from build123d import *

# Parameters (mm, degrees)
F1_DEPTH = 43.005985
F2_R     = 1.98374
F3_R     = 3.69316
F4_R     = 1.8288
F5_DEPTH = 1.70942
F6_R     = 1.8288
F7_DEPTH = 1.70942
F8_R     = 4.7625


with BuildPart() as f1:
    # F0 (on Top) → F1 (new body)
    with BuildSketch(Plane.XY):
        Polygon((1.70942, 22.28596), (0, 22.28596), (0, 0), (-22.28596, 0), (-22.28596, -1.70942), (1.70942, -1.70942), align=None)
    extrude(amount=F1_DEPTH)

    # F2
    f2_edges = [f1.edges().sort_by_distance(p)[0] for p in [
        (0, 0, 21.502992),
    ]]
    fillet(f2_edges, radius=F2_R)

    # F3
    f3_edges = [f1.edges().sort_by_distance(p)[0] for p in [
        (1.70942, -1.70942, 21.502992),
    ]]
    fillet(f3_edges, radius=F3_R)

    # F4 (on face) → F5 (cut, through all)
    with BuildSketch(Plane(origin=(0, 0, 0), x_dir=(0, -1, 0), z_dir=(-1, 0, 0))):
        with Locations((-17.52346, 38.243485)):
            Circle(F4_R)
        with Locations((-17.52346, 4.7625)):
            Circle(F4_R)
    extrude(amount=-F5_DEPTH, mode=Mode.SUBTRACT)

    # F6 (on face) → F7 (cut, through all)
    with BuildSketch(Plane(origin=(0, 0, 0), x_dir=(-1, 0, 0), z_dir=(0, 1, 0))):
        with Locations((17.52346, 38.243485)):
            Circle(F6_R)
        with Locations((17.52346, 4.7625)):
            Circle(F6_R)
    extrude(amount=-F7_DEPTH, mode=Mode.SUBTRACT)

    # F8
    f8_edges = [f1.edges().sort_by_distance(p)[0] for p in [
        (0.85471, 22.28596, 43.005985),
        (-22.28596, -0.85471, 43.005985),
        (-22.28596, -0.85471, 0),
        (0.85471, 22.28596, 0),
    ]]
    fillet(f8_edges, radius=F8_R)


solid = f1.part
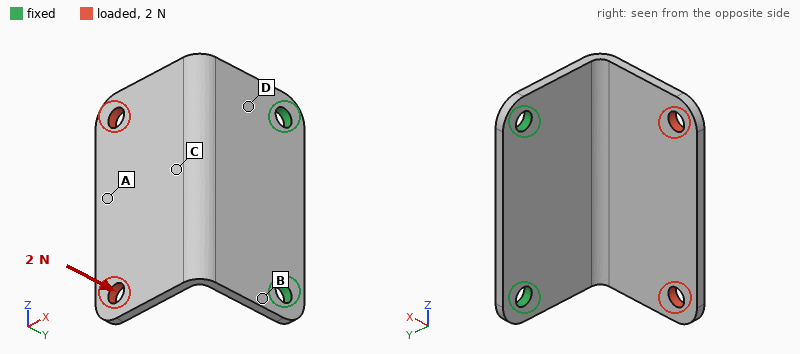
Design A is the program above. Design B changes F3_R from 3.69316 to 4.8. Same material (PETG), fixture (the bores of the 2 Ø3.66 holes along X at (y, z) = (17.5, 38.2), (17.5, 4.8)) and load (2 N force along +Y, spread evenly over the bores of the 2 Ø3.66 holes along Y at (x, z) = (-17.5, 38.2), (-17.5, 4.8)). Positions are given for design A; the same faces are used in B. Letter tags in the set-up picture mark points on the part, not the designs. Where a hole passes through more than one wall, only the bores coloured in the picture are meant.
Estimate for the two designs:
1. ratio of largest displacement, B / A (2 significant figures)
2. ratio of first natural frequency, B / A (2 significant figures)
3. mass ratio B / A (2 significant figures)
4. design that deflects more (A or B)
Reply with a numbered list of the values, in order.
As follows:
1. 1.1
2. 0.97
3. 0.97
4. B
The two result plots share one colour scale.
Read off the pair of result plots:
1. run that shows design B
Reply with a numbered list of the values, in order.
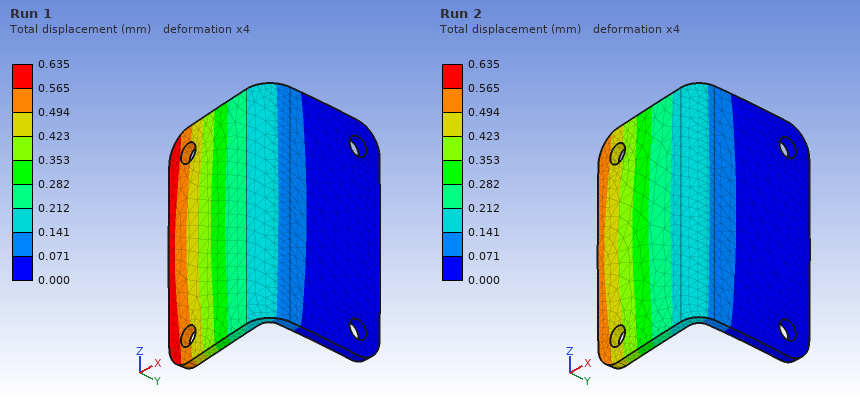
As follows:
1. Run 1
